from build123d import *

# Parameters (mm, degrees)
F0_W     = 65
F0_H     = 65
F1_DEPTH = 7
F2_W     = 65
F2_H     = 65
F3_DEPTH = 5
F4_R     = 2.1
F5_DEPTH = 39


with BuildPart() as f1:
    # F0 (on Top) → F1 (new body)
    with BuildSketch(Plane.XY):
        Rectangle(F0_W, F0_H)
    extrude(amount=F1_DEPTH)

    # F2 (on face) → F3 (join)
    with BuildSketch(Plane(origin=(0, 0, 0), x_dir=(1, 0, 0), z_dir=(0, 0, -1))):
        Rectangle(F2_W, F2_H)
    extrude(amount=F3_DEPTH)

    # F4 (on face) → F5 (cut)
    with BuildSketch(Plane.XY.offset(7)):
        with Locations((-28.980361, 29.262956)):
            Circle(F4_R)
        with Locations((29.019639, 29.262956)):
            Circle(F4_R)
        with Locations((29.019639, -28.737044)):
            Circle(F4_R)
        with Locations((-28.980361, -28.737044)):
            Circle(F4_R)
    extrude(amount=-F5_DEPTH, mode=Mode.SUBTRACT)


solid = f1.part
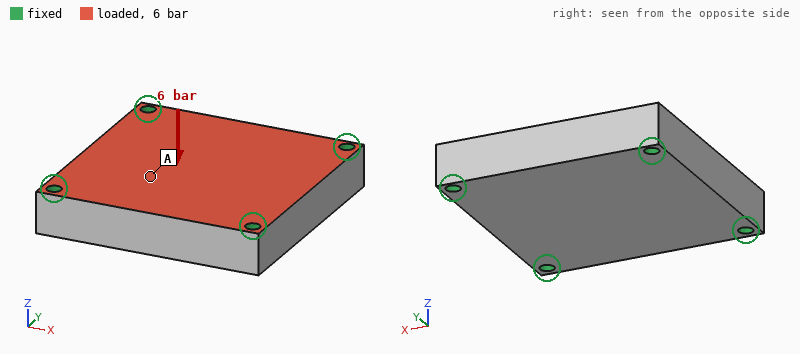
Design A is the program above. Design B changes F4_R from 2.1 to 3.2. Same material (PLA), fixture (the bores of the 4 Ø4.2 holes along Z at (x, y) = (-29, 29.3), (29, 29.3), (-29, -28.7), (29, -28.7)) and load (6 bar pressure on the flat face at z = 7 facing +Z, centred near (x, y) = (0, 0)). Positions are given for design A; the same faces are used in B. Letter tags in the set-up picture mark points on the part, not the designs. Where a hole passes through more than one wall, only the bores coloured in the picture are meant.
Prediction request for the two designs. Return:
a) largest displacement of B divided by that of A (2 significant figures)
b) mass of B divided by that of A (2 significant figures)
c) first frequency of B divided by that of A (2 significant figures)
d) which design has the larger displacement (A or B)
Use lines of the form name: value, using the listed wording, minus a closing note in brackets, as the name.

largest displacement of B divided by that of A: 0.84
mass of B divided by that of A: 0.98
first frequency of B divided by that of A: 1.1
which design has the larger displacement: A
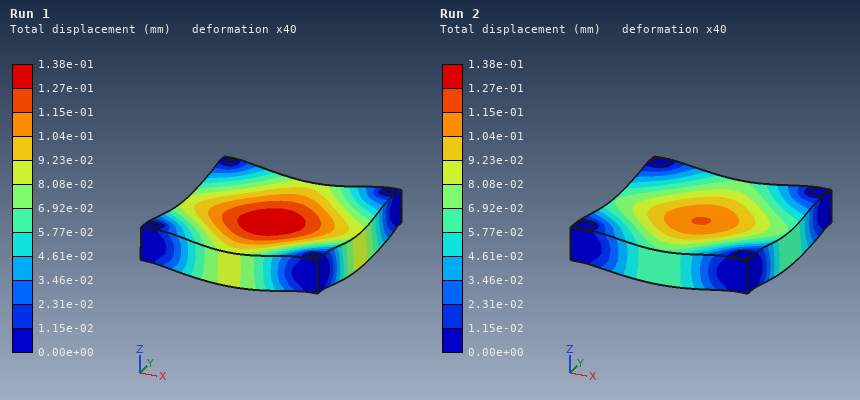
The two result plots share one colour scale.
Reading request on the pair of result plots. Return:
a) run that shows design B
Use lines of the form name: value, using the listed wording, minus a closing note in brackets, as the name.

run that shows design B: Run 2
